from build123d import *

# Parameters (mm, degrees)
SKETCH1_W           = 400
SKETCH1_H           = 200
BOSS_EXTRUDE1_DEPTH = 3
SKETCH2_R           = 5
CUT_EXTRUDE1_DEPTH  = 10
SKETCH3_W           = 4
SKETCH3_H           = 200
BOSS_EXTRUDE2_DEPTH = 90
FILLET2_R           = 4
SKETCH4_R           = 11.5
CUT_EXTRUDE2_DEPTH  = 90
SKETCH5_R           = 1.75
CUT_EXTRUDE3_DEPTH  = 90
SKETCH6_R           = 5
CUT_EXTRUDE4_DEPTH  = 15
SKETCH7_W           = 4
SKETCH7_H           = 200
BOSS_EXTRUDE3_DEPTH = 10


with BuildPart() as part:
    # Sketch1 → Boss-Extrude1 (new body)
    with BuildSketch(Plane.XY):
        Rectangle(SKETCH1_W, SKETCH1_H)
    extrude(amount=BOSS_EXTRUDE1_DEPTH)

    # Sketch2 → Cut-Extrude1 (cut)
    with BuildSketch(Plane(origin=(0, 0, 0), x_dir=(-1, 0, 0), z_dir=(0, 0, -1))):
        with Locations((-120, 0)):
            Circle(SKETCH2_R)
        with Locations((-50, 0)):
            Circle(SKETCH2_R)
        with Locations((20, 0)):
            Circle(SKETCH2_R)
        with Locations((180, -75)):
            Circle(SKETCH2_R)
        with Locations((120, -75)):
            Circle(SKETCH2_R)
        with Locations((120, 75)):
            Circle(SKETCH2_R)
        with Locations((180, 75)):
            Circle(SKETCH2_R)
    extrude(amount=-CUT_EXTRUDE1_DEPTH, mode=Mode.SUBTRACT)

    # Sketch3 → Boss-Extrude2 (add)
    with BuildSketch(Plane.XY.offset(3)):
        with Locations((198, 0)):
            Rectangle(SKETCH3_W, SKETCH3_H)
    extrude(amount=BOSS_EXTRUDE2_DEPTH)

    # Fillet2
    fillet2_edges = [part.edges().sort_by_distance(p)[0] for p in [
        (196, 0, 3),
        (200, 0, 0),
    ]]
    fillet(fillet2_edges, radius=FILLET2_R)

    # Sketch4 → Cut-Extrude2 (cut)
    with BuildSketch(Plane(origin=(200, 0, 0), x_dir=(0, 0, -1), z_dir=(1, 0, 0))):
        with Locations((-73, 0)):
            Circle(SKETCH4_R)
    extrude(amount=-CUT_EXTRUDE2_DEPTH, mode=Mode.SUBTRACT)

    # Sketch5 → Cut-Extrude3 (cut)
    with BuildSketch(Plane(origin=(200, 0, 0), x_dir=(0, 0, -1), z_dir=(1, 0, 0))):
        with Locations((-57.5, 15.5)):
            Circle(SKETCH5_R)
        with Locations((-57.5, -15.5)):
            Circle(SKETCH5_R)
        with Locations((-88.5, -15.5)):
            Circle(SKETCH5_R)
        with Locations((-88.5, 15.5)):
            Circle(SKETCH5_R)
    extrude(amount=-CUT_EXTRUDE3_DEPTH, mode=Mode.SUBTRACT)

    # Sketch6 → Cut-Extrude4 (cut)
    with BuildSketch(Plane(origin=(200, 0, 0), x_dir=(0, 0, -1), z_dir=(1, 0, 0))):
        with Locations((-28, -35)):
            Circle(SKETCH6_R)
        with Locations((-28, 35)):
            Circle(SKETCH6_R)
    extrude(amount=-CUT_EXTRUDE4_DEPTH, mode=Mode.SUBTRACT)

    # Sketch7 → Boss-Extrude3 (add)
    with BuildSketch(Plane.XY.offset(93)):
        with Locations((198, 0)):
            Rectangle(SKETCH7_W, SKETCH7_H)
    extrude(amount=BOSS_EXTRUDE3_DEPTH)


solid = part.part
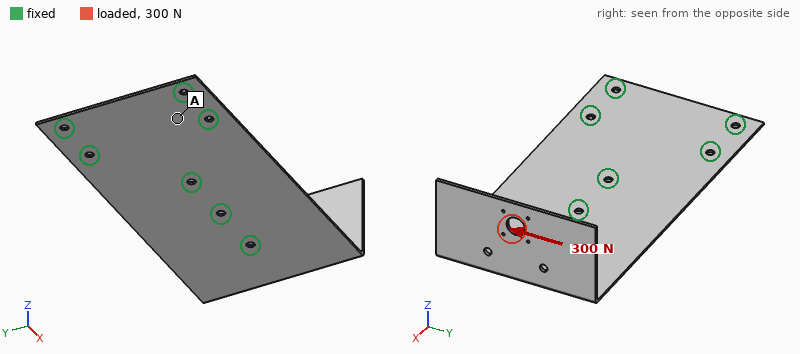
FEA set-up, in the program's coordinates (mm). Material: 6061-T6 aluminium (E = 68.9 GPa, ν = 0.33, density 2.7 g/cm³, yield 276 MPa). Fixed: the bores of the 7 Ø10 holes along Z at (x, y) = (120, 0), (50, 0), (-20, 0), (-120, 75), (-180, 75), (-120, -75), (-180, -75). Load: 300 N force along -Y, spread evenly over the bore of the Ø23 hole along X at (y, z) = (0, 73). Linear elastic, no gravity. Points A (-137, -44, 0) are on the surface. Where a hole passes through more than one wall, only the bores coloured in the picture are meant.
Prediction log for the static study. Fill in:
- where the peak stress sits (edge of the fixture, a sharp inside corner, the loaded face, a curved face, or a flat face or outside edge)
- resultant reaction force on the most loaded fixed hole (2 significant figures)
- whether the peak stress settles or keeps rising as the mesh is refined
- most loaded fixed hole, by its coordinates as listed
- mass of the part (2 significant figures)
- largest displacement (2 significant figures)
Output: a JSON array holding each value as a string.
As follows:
["edge of the fixture", "390 N", "keeps rising", "(120, 0)", "850 g", "4.5 mm"]
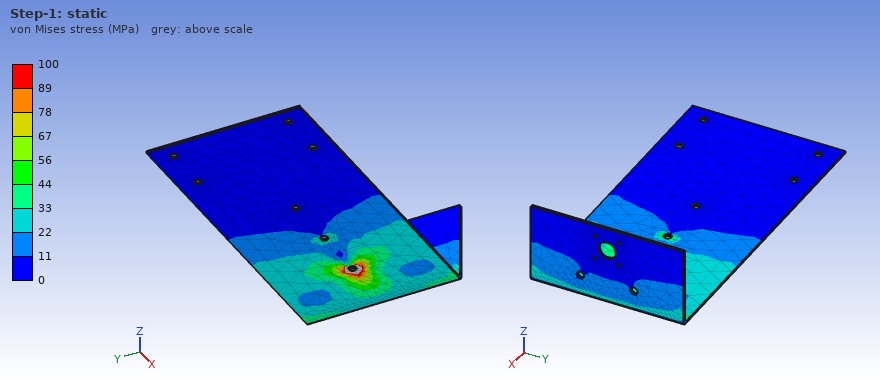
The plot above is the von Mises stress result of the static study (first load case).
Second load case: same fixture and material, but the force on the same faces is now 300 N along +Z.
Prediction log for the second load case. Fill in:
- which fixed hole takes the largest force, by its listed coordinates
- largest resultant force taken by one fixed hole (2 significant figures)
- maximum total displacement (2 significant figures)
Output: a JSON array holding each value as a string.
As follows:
["(120, 0)", "440 N", "4.2 mm"]
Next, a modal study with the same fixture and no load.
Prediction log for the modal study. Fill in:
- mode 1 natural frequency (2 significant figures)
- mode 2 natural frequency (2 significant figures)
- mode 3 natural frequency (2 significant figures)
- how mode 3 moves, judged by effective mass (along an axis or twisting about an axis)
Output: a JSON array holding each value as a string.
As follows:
["85 Hz", "99 Hz", "240 Hz", "along Z"]
